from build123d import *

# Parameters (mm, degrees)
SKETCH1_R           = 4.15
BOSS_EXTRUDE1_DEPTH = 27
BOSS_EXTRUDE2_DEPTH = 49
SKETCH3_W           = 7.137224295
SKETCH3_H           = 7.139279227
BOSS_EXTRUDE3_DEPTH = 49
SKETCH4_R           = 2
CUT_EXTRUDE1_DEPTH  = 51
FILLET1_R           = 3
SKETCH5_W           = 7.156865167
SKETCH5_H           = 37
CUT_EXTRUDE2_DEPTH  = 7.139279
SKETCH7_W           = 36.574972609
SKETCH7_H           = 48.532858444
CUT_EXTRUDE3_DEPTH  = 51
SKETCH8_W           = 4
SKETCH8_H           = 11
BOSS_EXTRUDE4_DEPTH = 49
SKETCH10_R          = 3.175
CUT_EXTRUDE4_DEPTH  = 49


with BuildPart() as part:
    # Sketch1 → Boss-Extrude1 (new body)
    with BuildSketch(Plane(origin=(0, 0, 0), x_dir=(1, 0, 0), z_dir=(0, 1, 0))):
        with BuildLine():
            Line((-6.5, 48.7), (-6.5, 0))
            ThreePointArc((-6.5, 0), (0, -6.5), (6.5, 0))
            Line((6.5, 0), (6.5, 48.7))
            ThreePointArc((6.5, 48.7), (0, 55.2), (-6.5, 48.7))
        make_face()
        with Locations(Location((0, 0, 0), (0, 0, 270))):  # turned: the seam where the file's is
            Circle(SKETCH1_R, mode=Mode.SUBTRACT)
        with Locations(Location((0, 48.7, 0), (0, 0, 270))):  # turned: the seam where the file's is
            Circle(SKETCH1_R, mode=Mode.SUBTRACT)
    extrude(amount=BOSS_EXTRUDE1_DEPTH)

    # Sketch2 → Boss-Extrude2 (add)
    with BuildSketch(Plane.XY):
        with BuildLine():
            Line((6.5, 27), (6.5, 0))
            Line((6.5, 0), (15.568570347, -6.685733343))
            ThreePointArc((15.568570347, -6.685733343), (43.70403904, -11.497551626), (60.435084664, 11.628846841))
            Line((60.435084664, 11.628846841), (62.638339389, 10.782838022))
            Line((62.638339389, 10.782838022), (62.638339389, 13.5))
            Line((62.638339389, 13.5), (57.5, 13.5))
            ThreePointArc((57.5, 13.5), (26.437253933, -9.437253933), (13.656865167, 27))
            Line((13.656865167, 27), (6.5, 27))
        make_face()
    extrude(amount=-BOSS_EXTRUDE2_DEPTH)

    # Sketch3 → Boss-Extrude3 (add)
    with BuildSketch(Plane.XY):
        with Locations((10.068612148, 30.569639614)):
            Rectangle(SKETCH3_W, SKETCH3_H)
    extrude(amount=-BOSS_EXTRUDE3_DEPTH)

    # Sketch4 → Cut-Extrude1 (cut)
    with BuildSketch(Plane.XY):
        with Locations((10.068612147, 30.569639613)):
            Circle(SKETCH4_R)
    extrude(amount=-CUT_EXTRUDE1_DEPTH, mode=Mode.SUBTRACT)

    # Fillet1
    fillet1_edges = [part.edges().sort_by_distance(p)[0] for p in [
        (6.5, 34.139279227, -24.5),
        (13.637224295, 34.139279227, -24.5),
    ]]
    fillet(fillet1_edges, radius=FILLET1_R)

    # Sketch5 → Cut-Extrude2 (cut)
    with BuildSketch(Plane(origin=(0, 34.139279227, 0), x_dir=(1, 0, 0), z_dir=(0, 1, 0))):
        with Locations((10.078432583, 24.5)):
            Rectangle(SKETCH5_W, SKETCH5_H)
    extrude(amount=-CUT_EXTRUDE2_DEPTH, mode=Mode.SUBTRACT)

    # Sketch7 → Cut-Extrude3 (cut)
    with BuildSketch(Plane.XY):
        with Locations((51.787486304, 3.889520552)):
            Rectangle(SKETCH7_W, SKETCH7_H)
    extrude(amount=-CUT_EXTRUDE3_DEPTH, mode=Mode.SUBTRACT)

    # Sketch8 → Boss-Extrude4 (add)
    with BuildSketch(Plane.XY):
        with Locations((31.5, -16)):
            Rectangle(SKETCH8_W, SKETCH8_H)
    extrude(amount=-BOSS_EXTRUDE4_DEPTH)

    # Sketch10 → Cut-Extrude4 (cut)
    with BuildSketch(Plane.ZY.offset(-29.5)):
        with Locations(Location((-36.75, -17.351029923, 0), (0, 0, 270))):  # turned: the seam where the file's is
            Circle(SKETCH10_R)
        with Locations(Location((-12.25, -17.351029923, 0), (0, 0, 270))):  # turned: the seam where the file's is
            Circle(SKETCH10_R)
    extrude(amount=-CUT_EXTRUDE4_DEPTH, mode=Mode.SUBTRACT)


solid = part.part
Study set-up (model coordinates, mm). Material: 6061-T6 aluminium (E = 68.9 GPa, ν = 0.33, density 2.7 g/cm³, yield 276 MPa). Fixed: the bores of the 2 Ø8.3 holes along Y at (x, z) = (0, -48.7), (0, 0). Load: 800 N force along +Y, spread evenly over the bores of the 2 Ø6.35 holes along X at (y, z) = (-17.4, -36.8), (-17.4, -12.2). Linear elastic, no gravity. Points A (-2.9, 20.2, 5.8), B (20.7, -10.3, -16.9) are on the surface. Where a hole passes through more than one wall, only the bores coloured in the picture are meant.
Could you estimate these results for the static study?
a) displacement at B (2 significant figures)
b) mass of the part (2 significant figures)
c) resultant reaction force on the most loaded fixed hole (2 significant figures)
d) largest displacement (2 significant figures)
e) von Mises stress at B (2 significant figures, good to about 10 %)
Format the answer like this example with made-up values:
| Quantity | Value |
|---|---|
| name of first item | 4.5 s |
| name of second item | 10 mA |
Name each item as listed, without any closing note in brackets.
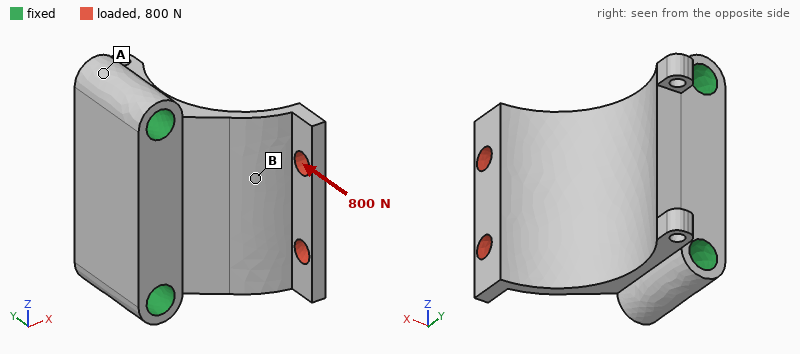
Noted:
| Quantity | Value |
|---|---|
| displacement at B | 0.13 mm |
| mass of the part | 80 g |
| resultant reaction force on the most loaded fixed hole | 400 N |
| largest displacement | 0.49 mm |
| von Mises stress at B | 93 MPa |
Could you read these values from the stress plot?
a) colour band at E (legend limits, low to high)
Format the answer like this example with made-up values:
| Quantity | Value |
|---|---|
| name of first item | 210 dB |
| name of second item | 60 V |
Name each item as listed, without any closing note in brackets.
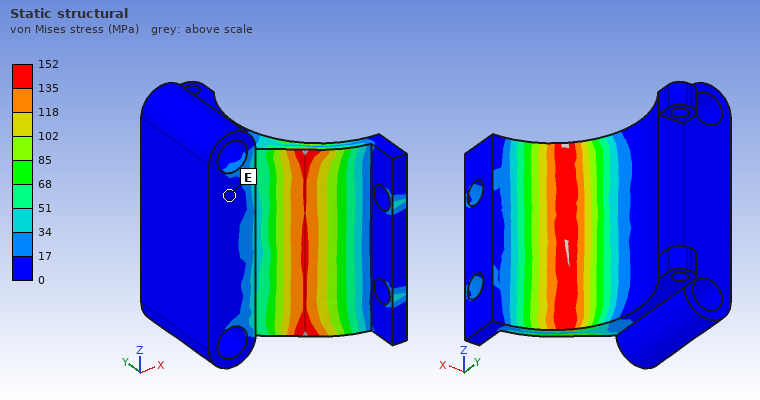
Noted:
| Quantity | Value |
|---|---|
| colour band at E | 0 to 17 MPa |
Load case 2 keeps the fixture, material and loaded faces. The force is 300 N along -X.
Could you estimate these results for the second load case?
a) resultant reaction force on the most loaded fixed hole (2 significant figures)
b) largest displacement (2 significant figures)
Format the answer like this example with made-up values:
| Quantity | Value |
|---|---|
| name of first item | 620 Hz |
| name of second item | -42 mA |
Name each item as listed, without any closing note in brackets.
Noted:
| Quantity | Value |
|---|---|
| resultant reaction force on the most loaded fixed hole | 160 N |
| largest displacement | 0.16 mm |
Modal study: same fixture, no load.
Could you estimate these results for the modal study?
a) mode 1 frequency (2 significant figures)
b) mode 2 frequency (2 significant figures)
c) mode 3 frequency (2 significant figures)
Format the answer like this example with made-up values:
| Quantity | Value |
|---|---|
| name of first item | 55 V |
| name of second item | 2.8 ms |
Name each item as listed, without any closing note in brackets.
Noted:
| Quantity | Value |
|---|---|
| mode 1 frequency | 2600 Hz |
| mode 2 frequency | 4500 Hz |
| mode 3 frequency | 14 kHz |
